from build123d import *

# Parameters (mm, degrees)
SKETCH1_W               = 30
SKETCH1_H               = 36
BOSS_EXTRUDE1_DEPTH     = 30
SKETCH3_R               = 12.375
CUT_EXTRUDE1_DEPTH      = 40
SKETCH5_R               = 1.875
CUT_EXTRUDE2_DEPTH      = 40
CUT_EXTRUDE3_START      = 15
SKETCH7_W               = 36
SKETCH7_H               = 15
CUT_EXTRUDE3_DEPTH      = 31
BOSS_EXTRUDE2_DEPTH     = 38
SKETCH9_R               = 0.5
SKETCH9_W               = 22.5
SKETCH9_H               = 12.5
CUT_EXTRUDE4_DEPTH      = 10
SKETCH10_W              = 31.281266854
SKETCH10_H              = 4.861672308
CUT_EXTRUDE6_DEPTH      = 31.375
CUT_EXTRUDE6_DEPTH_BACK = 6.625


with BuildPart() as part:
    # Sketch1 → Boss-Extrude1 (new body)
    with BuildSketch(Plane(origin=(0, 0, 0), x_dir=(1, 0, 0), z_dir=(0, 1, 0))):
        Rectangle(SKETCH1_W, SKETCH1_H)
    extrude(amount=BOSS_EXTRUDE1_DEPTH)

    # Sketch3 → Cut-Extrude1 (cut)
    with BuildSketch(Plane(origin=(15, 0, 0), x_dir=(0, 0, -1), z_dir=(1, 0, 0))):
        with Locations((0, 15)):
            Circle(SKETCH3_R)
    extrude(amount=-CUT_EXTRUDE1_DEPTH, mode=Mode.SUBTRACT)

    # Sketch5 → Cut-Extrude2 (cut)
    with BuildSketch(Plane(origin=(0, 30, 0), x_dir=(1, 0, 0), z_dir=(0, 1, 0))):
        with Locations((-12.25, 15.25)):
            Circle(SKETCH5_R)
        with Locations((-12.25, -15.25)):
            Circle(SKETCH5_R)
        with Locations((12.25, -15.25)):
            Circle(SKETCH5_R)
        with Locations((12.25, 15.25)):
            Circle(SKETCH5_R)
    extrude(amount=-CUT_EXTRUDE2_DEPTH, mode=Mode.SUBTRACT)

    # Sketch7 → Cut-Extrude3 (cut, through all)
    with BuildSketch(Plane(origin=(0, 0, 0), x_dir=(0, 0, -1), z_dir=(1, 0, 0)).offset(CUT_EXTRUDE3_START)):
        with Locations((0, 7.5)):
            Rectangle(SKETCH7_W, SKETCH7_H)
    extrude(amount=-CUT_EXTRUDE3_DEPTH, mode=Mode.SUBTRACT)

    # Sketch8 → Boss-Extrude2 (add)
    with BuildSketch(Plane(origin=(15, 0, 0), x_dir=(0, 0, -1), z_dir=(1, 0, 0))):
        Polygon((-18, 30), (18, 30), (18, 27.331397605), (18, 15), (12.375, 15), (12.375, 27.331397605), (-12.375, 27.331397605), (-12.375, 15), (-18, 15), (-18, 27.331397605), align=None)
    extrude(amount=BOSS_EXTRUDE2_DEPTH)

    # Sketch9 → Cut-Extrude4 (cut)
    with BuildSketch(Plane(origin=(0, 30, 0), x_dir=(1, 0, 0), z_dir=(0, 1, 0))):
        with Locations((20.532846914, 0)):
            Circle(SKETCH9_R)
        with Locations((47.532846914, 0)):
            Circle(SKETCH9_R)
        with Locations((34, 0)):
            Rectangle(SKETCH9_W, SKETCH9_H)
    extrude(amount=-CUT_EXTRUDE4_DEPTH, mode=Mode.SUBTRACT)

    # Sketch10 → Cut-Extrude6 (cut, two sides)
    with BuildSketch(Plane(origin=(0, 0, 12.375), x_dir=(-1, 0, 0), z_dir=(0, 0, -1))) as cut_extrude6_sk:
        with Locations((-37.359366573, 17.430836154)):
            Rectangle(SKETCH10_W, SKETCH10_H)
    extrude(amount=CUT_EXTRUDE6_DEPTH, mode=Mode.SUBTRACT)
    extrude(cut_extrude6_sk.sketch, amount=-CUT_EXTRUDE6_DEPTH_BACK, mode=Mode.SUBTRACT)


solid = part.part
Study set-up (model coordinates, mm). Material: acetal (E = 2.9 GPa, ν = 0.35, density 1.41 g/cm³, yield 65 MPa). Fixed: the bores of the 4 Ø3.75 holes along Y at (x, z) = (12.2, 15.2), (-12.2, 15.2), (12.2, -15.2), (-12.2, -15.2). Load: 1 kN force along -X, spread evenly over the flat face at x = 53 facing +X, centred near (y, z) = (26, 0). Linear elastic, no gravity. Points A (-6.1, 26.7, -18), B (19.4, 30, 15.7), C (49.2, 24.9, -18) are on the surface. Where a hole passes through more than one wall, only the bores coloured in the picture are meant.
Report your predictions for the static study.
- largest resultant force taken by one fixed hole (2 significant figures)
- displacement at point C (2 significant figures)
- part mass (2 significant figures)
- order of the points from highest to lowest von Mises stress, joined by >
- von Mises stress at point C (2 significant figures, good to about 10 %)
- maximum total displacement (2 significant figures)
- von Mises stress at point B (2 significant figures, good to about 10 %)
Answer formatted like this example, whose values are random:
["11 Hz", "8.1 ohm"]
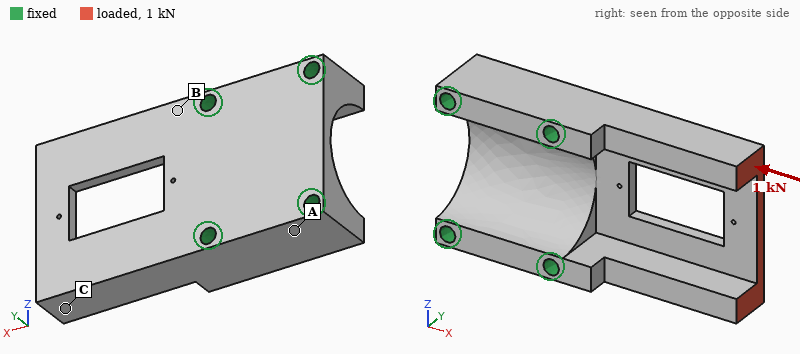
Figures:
["470 N", "0.12 mm", "21 g", "B > C > A", "4.9 MPa", "0.21 mm", "9.4 MPa"]
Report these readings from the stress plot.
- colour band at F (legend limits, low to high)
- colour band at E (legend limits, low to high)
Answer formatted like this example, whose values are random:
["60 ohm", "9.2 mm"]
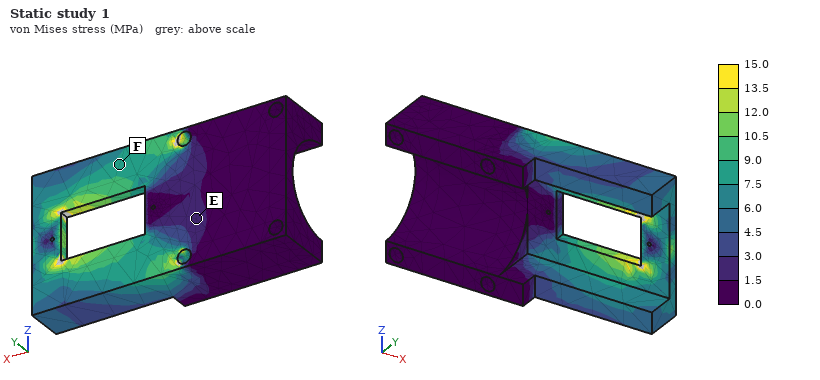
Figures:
["7.5 to 9.0 MPa", "1.5 to 3.0 MPa"]
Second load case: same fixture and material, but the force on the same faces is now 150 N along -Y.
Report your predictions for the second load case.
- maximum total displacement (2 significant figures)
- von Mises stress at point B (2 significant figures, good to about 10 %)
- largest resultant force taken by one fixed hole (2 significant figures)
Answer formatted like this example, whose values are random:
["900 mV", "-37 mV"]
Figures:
["0.88 mm", "13 MPa", "100 N"]
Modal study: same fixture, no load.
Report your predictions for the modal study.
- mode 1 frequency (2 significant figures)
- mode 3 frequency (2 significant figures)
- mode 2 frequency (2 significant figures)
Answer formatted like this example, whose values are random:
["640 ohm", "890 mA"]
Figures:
["1600 Hz", "2400 Hz", "1600 Hz"]
